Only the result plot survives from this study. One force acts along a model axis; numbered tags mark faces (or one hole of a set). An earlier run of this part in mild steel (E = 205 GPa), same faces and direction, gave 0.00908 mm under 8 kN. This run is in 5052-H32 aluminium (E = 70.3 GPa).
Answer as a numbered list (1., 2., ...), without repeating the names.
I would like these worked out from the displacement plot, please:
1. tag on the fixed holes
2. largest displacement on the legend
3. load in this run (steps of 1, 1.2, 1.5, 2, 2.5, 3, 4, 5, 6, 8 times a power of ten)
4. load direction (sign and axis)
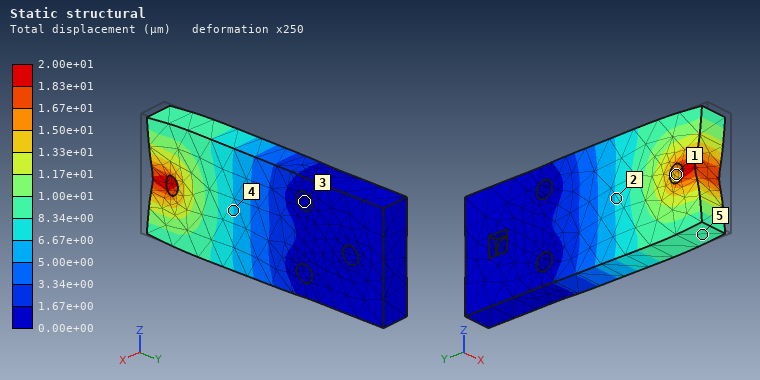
1. 3
2. 2.00e+01 µm
3. 6 kN
4. +Y
